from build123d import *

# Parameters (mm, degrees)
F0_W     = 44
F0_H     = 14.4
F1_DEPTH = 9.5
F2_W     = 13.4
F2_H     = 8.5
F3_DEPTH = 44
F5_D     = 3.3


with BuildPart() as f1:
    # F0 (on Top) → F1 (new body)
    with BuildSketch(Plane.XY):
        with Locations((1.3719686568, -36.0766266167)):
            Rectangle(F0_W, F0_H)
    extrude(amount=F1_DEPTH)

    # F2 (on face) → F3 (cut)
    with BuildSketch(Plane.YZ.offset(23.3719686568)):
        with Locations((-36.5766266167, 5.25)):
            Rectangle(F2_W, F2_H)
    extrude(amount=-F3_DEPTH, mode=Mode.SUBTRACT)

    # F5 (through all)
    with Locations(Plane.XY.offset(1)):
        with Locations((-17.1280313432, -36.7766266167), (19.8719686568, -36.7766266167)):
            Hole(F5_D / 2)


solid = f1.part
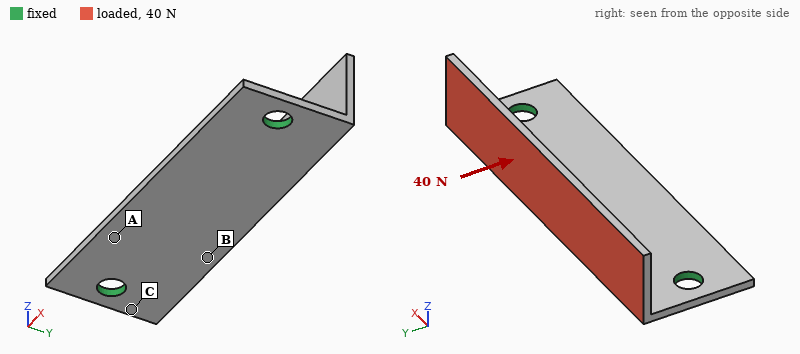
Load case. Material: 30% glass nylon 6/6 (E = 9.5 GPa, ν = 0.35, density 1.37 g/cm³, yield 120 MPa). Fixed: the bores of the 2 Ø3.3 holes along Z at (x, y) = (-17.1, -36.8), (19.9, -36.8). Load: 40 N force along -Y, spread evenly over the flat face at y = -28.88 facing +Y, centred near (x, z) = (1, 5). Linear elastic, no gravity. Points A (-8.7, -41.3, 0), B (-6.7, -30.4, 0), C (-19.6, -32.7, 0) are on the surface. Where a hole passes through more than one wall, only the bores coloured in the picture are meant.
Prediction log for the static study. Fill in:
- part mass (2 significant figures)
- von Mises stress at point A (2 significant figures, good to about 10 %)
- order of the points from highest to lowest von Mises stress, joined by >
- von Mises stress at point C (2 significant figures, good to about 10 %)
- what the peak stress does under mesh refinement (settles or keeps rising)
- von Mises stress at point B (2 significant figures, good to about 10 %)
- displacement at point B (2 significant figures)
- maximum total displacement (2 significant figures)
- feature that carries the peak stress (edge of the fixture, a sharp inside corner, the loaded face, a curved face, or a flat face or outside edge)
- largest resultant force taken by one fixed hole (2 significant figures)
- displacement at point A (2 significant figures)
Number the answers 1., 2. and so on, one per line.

1. 1.4 g
2. 8.0 MPa
3. C > B > A
4. 33 MPa
5. keeps rising
6. 19 MPa
7. 0.11 mm
8. 0.49 mm
9. edge of the fixture
10. 20 N
11. 0.099 mm
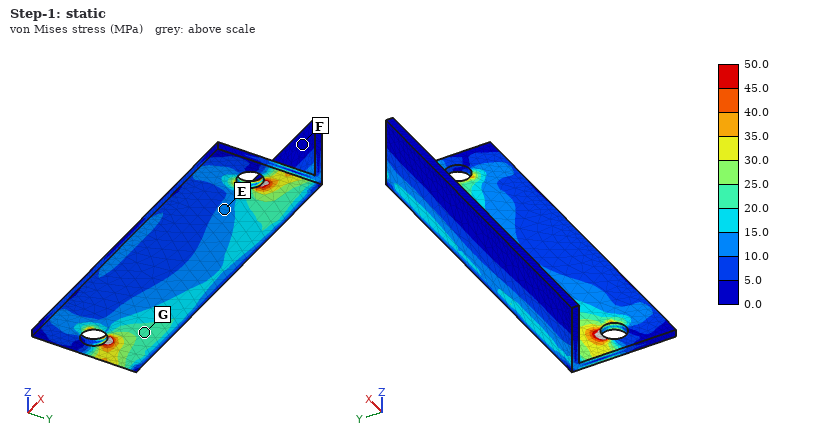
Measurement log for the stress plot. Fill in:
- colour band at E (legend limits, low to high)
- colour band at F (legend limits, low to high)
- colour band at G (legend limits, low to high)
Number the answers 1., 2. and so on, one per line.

1. 10.0 to 15.0 MPa
2. 0.0 to 5.0 MPa
3. 20.0 to 25.0 MPa
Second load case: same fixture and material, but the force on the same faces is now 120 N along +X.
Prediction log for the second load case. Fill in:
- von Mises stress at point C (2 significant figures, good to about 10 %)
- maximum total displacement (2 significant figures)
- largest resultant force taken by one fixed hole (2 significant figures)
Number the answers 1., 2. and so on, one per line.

1. 20 MPa
2. 0.19 mm
3. 66 N
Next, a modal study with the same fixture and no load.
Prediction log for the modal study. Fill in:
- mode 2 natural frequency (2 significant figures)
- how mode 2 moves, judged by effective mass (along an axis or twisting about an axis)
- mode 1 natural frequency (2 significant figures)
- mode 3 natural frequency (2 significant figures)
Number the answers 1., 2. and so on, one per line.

1. 2900 Hz
2. along Z
3. 1900 Hz
4. 3100 Hz
